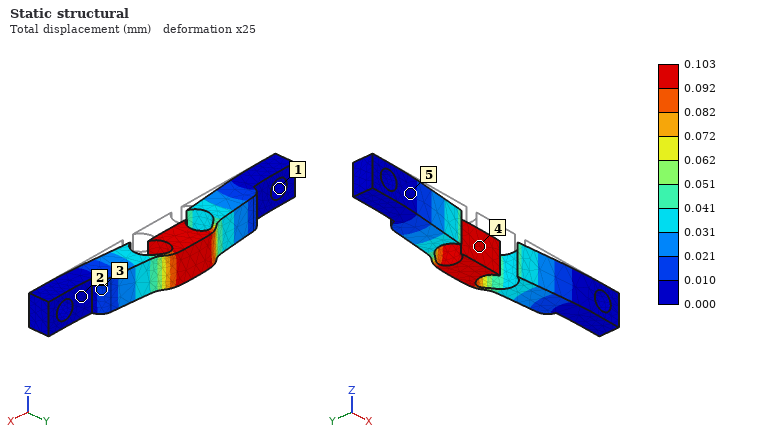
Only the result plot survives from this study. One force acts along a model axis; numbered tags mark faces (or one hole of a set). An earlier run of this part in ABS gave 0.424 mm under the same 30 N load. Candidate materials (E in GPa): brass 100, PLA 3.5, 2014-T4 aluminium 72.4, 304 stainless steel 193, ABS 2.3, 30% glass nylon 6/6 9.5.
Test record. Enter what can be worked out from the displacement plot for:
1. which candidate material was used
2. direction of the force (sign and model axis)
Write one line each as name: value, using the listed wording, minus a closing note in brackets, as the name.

which candidate material was used: 30% glass nylon 6/6
direction of the force: +Y
